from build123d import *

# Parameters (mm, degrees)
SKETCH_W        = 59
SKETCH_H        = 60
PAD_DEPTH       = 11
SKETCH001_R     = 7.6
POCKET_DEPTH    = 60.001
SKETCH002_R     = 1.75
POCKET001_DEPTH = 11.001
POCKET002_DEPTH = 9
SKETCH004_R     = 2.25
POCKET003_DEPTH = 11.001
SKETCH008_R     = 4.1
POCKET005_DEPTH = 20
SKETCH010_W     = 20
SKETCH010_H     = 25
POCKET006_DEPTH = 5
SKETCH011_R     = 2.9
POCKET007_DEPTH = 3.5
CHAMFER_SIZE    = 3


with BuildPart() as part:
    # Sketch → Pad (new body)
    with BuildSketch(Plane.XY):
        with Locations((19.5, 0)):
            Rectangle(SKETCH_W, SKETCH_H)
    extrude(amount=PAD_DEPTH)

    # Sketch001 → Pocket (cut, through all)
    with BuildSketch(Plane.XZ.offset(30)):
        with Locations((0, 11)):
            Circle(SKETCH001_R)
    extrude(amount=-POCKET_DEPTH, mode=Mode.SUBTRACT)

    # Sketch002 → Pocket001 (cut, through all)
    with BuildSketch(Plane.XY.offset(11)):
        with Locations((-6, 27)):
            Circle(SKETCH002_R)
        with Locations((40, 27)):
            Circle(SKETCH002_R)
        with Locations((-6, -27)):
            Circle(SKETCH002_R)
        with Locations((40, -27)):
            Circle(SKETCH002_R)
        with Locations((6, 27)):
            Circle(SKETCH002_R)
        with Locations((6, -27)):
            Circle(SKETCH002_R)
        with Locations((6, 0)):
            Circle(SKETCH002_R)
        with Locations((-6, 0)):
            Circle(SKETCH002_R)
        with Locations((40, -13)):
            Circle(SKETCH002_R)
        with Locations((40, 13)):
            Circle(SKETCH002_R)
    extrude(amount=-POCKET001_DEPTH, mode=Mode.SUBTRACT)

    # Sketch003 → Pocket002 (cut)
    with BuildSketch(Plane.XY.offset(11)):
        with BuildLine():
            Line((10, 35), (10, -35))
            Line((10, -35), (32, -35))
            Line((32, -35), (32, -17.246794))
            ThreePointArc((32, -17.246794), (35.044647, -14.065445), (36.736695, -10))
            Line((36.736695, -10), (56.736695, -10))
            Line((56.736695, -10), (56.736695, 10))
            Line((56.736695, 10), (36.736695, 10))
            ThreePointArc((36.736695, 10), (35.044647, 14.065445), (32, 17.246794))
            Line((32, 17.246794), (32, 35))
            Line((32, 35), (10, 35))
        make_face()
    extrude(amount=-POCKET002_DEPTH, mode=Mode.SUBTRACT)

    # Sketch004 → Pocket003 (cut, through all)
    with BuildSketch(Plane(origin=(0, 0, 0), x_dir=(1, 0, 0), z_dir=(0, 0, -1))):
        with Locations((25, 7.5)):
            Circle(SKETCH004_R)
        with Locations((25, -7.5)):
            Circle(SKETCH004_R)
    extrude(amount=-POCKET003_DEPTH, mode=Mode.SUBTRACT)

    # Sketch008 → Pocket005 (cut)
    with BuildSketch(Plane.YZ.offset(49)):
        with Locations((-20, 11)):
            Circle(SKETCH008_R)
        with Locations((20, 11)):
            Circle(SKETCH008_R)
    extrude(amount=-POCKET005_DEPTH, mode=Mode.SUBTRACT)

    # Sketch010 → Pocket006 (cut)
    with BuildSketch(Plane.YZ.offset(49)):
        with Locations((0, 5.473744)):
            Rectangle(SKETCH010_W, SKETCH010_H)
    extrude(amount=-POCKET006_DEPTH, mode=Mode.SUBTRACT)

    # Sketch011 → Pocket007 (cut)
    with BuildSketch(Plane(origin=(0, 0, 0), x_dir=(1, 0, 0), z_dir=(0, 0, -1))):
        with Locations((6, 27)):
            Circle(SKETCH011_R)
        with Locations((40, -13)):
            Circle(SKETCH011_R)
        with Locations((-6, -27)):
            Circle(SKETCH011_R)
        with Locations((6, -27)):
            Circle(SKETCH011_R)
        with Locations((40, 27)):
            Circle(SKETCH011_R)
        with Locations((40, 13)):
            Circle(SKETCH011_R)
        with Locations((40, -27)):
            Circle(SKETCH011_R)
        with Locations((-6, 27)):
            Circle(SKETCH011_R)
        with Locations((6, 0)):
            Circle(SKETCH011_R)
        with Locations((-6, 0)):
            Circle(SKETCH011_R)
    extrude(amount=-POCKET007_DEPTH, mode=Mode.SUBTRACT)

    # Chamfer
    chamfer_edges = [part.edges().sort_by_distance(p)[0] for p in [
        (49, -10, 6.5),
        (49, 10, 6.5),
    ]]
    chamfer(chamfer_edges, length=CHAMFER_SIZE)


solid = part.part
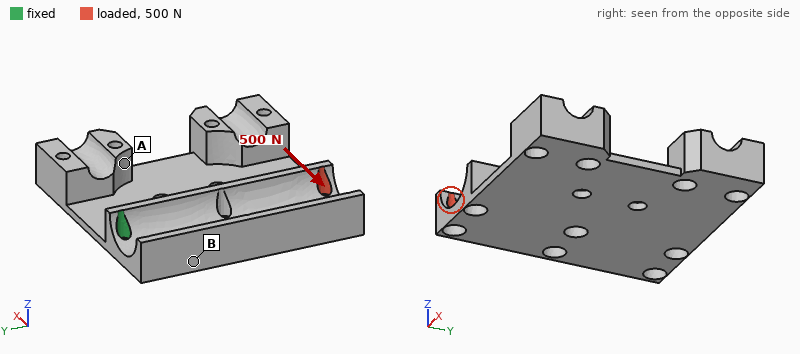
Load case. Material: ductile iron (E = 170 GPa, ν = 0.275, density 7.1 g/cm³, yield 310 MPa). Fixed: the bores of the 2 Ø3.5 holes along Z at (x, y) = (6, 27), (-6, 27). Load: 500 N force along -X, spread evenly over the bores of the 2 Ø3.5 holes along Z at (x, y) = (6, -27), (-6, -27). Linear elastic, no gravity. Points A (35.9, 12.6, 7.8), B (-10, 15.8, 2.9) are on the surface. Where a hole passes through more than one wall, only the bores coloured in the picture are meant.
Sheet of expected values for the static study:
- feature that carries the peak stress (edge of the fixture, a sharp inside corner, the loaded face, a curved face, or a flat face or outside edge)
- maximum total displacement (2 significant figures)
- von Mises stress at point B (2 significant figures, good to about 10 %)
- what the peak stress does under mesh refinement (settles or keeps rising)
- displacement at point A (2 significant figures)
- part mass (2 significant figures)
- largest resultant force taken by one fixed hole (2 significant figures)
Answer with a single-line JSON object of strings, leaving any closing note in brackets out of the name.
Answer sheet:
{"feature that carries the peak stress": "edge of the fixture", "maximum total displacement": "0.12 mm", "von Mises stress at point B": "38 MPa", "what the peak stress does under mesh refinement": "keeps rising", "displacement at point A": "0.048 mm", "part mass": "110 g", "largest resultant force taken by one fixed hole": "1.7 kN"}
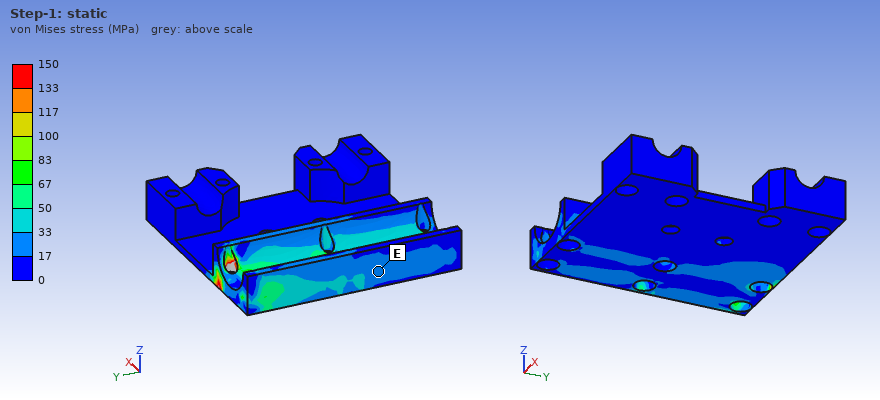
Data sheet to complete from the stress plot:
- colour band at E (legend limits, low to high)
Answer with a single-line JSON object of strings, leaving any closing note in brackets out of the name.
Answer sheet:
{"colour band at E": "17 to 33 MPa"}
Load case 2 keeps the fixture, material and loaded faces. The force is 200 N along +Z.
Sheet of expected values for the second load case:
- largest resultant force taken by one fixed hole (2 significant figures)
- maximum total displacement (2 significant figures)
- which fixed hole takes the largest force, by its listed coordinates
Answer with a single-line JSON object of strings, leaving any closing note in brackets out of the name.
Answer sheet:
{"largest resultant force taken by one fixed hole": "110 N", "maximum total displacement": "95 µm", "which fixed hole takes the largest force, by its listed coordinates": "(-6, 27)"}
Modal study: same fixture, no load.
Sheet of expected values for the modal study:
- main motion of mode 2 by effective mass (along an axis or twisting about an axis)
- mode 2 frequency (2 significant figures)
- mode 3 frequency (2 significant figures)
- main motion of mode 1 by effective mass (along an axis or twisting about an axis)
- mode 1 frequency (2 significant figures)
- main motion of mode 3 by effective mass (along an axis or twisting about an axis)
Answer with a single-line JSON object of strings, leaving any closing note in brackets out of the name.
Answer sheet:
{"main motion of mode 2 by effective mass": "twisting about X", "mode 2 frequency": "910 Hz", "mode 3 frequency": "1900 Hz", "main motion of mode 1 by effective mass": "along Z", "mode 1 frequency": "510 Hz", "main motion of mode 3 by effective mass": "along Z"}
